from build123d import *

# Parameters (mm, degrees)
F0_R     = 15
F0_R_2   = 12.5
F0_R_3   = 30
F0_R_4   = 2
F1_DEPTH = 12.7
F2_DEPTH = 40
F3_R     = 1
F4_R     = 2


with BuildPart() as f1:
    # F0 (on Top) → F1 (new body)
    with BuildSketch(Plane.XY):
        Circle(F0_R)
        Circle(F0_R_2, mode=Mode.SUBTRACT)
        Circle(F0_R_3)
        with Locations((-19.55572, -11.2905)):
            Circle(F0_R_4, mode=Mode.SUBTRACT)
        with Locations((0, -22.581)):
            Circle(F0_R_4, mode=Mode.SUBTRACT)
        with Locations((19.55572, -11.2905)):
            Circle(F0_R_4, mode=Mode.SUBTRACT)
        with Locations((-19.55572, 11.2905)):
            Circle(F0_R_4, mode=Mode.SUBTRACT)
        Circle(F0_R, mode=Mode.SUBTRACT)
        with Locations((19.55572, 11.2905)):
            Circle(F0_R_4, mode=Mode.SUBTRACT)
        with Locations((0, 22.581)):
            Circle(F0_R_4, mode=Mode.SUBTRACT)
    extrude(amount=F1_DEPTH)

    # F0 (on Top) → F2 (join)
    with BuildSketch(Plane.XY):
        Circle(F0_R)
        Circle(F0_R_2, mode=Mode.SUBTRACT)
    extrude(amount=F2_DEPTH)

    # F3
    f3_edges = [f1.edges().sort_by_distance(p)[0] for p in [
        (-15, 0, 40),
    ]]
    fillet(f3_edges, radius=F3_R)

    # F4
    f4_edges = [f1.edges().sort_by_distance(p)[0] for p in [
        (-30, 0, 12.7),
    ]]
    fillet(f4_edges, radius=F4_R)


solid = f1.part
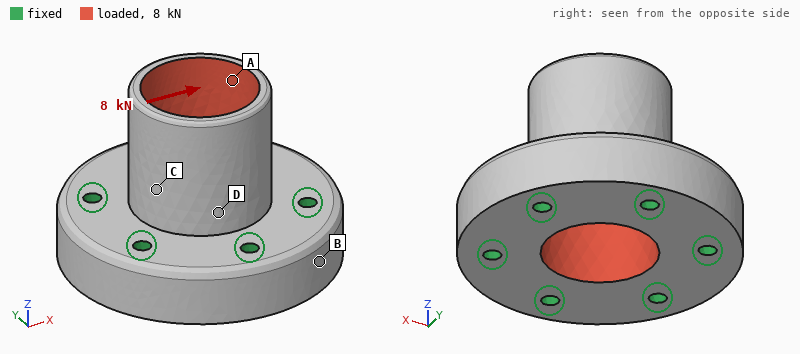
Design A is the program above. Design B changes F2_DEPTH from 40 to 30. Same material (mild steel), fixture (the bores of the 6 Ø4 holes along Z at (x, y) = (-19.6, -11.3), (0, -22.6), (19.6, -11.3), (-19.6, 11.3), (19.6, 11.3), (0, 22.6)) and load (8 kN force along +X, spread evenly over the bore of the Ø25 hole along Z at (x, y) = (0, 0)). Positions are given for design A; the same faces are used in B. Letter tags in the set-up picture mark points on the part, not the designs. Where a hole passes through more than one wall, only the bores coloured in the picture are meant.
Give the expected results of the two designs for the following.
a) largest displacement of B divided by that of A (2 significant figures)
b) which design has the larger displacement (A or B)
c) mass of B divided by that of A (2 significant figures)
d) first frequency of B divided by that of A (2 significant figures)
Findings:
0.52
A
0.94
1.5
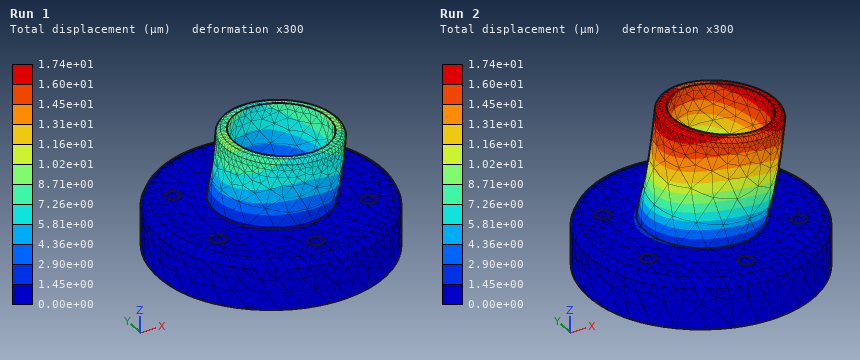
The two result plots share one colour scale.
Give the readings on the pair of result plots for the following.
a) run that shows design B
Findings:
Run 1
